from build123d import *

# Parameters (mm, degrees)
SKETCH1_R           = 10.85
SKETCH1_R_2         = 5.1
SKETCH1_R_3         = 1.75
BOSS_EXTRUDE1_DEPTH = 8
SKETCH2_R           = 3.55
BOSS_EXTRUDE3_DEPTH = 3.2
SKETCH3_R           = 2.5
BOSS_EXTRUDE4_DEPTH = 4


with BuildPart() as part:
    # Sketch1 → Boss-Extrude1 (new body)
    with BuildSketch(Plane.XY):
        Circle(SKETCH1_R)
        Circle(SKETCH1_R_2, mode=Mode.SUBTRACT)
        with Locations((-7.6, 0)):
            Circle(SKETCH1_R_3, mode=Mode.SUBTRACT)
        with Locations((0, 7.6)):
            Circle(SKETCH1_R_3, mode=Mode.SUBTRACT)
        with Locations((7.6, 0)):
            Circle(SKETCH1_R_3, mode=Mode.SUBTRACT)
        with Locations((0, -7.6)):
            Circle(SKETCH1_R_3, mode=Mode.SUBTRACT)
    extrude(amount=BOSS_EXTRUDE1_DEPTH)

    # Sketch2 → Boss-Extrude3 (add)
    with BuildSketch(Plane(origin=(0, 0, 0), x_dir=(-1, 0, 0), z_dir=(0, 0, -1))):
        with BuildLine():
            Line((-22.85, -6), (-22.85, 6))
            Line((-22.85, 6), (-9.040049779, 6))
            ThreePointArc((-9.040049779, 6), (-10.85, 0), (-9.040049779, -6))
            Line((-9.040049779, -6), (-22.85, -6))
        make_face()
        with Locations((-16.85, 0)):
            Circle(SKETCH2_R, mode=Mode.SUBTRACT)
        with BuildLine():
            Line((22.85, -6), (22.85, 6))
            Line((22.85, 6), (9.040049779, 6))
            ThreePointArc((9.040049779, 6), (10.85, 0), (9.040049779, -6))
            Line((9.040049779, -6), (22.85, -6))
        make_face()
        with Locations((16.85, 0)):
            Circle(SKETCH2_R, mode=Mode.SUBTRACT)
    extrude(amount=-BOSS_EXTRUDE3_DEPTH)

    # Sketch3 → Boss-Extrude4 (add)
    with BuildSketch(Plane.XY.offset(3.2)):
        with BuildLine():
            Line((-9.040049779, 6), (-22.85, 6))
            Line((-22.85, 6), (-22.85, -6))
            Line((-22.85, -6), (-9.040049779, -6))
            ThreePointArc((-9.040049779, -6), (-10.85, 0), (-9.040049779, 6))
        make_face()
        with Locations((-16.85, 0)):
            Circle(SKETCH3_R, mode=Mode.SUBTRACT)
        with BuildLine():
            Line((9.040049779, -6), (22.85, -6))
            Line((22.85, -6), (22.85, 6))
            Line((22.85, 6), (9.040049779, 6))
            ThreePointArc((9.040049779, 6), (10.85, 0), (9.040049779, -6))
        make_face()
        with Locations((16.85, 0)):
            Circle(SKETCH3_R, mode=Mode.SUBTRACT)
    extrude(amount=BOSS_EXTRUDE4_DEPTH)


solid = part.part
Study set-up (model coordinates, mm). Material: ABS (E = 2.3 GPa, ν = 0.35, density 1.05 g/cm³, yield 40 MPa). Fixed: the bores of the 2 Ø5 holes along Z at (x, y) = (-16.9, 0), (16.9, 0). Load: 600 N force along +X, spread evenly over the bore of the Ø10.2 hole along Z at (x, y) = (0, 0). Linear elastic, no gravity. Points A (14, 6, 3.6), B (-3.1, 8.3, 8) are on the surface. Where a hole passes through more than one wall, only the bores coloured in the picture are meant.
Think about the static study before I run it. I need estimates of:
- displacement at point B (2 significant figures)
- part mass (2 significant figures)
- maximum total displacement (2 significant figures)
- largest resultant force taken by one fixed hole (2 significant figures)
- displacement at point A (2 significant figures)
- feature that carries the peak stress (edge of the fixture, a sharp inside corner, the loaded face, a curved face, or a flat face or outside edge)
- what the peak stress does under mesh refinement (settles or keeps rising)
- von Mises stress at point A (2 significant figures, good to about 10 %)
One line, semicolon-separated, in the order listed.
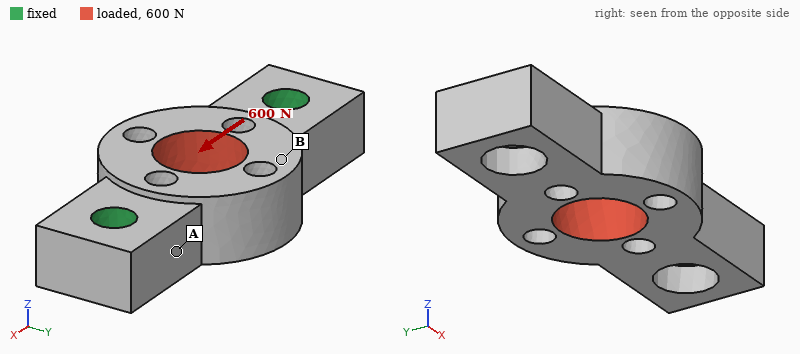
25 µm; 3.9 g; 35 µm; 300 N; 13 µm; edge of the fixture; keeps rising; 2.8 MPa
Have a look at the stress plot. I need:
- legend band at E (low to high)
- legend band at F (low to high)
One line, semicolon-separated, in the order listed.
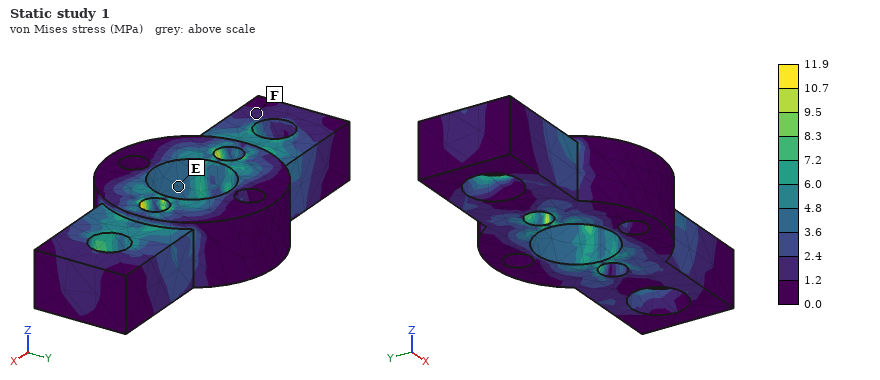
3.6 to 4.8 MPa; 1.2 to 2.4 MPa
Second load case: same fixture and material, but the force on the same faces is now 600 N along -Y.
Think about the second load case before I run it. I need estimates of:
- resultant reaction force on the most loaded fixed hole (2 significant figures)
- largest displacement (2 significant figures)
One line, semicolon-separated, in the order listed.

300 N; 0.13 mm
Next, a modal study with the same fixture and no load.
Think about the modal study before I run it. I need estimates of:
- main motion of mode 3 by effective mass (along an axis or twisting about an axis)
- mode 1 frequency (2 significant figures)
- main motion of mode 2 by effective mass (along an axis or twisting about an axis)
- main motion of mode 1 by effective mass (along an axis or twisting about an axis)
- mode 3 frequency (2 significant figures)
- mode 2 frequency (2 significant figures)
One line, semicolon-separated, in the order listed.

along Y; 5400 Hz; along Z; twisting about X; 9300 Hz; 5700 Hz
